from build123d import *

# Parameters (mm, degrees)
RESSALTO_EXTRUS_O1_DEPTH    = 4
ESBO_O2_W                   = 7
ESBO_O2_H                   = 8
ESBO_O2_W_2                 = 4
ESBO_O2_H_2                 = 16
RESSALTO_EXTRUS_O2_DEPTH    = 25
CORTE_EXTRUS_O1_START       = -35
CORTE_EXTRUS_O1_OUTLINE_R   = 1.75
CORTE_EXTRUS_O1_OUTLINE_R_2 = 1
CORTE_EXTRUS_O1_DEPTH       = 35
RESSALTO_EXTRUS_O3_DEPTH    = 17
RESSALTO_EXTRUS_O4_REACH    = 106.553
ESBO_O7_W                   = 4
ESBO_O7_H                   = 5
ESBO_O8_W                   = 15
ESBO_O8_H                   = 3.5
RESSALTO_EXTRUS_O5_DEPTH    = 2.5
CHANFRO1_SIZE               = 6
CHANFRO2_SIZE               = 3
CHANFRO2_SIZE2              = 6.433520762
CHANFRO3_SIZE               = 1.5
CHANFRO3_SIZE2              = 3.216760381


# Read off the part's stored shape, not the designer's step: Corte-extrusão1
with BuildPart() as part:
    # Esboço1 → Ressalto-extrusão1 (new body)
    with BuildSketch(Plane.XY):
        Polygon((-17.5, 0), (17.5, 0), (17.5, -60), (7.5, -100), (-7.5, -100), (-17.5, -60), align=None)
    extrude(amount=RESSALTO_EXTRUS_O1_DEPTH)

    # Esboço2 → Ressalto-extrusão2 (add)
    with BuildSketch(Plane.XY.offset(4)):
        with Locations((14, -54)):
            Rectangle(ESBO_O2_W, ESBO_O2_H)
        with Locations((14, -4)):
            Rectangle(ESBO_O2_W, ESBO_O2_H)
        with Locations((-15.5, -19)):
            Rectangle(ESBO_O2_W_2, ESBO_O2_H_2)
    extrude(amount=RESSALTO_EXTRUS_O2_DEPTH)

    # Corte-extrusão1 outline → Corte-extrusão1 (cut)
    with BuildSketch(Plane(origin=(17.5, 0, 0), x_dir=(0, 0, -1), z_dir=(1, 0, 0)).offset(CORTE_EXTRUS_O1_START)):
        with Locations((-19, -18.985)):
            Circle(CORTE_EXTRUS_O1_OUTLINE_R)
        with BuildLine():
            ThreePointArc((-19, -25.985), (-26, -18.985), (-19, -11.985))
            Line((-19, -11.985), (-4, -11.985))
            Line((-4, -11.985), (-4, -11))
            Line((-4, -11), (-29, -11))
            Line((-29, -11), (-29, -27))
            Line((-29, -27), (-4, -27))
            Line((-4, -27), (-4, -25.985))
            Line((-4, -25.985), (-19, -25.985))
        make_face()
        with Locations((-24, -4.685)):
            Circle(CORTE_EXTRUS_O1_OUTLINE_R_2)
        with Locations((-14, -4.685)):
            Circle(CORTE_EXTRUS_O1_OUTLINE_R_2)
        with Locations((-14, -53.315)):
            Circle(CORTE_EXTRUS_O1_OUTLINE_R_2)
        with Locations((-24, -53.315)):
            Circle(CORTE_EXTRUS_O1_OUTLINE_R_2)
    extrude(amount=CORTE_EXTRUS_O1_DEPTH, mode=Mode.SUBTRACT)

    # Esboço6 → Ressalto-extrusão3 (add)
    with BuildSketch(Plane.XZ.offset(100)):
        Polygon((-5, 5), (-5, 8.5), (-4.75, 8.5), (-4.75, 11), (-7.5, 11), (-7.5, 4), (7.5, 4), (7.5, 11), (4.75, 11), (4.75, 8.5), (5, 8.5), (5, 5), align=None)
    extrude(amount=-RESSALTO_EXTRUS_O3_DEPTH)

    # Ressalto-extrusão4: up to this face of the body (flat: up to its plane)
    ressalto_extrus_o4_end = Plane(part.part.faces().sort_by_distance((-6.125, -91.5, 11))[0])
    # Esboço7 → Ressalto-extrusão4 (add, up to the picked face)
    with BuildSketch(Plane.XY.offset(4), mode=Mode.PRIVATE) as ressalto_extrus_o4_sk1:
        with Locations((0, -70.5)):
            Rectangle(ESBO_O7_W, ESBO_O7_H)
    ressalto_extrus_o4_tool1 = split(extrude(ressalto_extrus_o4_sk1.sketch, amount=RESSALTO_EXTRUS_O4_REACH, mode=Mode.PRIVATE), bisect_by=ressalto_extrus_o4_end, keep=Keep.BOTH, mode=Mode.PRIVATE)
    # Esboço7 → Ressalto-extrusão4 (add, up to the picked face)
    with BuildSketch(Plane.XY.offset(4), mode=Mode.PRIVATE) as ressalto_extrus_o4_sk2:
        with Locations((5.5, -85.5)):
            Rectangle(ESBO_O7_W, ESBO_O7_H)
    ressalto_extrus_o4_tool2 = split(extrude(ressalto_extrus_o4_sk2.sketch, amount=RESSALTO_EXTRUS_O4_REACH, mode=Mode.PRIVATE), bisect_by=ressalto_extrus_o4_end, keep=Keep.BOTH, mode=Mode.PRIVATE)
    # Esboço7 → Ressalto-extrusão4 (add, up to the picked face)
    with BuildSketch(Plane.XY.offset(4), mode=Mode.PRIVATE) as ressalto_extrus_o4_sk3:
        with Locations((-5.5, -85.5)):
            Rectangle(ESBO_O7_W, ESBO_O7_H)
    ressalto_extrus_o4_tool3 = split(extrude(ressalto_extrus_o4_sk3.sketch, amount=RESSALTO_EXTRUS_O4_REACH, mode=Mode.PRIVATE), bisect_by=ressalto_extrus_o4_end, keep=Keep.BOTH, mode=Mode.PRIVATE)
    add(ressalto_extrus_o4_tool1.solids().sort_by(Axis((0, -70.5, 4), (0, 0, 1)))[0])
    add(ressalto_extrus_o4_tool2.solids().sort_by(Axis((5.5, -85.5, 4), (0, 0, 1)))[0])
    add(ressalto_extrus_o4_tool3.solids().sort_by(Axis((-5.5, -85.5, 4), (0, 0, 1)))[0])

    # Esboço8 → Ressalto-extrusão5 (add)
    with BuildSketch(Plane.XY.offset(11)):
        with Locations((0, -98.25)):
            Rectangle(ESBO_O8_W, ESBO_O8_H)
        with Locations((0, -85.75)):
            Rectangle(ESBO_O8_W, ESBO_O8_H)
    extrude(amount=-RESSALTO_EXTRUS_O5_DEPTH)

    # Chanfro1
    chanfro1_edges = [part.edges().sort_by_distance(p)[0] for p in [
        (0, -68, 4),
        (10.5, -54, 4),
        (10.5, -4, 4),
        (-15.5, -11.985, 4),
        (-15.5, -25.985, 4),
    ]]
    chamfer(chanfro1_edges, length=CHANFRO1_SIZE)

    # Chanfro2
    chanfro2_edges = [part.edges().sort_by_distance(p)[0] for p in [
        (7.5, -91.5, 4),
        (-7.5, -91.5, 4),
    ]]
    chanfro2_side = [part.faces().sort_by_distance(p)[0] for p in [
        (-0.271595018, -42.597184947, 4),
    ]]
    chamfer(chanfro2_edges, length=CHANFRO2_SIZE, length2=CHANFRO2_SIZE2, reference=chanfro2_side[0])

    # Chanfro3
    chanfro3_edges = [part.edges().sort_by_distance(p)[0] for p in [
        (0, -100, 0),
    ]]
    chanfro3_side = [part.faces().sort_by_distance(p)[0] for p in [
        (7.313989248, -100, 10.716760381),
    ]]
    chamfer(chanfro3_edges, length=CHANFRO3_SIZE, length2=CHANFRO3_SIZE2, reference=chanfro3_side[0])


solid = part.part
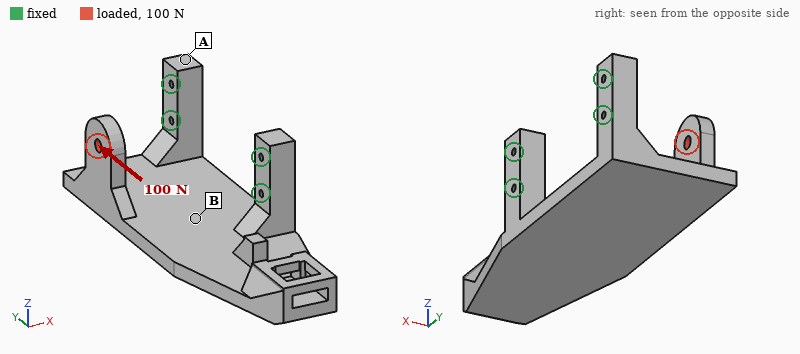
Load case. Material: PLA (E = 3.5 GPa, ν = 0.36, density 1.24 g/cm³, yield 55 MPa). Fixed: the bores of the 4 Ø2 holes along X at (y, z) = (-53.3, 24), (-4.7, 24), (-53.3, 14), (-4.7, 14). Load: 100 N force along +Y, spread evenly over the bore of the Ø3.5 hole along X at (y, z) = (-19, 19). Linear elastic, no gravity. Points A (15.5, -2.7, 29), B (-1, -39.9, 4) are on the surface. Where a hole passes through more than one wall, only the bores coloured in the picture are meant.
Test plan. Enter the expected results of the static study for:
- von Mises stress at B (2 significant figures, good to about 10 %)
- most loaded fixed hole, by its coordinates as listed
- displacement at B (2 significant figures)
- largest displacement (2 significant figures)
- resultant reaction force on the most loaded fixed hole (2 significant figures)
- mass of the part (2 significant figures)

5.4 MPa
(-4.7, 14)
0.18 mm
0.83 mm
120 N
22 g
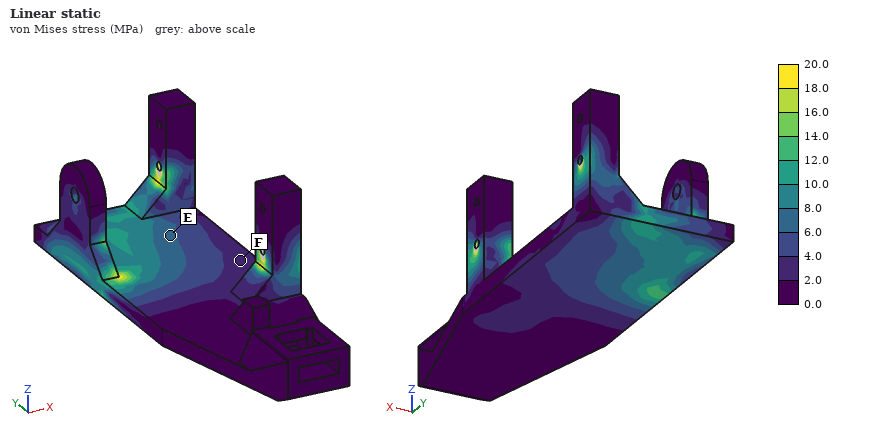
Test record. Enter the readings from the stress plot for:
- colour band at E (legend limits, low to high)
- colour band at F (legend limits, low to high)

6.0 to 8.0 MPa
2.0 to 4.0 MPa
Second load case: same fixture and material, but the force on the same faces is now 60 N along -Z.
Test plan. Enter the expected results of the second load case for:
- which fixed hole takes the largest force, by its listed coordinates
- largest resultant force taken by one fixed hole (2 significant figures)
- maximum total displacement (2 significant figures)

(-4.7, 14)
46 N
0.99 mm
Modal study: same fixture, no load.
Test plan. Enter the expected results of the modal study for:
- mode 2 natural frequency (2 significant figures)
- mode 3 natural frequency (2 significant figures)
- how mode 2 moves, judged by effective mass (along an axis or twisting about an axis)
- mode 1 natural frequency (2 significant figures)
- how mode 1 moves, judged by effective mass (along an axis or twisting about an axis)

670 Hz
1000 Hz
along Z
420 Hz
along Z
